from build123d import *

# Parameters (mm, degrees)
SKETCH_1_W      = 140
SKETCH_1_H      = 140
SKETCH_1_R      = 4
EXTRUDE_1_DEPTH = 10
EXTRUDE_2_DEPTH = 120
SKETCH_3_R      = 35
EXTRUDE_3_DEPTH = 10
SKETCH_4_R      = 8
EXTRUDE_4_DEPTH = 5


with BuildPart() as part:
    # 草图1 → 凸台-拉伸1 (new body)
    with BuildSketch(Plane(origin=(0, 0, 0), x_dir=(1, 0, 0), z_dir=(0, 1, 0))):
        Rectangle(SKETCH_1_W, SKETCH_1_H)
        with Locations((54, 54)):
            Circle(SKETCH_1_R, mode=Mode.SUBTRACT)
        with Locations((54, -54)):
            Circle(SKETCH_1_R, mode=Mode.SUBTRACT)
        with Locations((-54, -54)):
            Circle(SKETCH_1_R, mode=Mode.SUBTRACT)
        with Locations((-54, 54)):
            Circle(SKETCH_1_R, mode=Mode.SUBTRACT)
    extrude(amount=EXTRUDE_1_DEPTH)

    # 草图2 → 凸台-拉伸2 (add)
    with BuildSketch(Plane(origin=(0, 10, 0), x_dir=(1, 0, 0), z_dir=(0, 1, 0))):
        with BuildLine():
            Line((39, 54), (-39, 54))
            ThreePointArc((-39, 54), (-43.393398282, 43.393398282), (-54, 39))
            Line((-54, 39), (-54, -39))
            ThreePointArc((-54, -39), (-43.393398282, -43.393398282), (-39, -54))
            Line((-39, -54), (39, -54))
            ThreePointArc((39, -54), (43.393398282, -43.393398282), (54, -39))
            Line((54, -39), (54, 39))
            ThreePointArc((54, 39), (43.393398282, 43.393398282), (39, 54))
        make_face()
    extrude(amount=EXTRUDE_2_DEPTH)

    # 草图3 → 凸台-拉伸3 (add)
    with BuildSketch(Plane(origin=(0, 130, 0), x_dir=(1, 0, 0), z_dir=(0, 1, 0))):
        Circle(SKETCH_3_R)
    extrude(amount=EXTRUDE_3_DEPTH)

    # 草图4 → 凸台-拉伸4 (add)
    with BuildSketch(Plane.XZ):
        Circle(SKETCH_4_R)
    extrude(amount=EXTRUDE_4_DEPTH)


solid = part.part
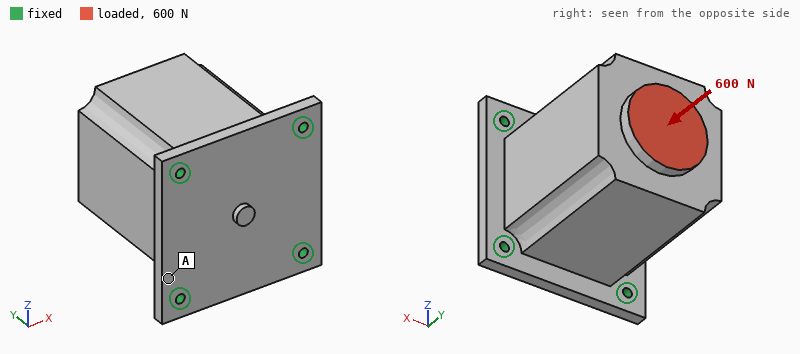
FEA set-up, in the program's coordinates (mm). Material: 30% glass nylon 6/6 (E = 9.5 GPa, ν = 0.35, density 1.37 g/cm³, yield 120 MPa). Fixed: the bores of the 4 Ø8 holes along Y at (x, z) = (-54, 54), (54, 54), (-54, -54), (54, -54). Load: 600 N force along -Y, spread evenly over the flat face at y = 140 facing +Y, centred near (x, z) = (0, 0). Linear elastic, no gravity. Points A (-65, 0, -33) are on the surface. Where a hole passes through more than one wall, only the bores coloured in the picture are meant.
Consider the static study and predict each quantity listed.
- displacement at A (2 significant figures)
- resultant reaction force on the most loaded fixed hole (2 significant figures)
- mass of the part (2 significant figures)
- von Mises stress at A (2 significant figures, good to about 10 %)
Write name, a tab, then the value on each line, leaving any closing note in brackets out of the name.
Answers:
displacement at A	3.8 µm
resultant reaction force on the most loaded fixed hole	160 N
mass of the part	2.1 kg
von Mises stress at A	0.37 MPa
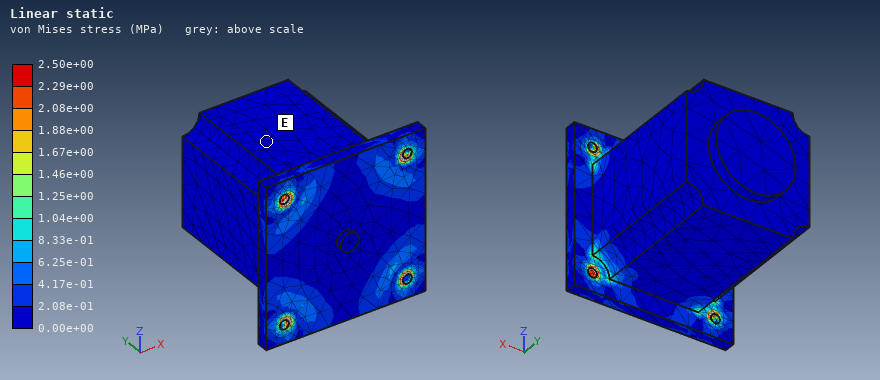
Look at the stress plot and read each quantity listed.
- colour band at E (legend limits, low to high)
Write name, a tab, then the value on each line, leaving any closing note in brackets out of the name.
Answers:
colour band at E	0.00e+00 to 2.08e-01 MPa
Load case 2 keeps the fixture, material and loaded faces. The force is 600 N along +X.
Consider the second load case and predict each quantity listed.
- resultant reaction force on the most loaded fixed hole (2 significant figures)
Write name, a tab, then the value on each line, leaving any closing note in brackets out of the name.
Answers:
resultant reaction force on the most loaded fixed hole	450 N
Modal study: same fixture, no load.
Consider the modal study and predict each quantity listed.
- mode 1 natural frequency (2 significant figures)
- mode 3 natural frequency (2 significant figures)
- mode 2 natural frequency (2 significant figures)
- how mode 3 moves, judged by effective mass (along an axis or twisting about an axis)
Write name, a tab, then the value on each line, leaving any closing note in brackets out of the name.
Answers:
mode 1 natural frequency	690 Hz
mode 3 natural frequency	1100 Hz
mode 2 natural frequency	690 Hz
how mode 3 moves, judged by effective mass	along Y
